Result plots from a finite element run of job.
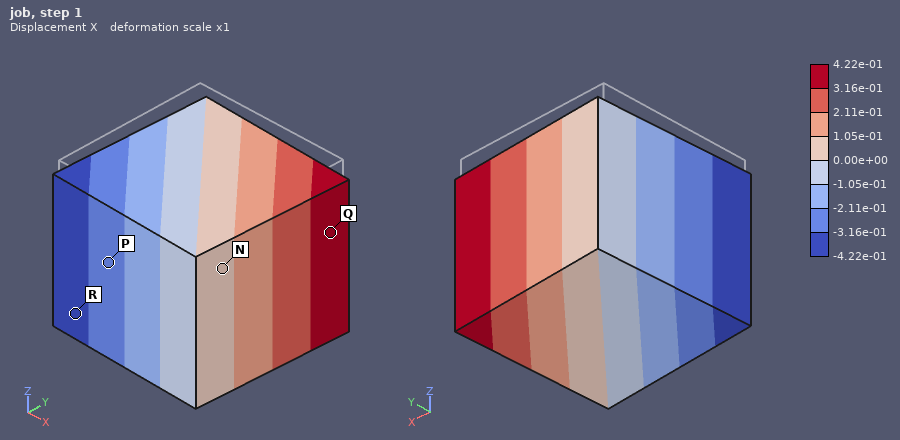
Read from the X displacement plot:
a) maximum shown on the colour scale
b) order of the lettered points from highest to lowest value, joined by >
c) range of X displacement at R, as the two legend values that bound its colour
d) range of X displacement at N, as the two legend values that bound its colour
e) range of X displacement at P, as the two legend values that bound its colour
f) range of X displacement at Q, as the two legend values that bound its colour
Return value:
4.22e-01
Q > N > P > R
-4.22e-01 to -3.16e-01
0.00e+00 to 1.05e-01
-3.16e-01 to -2.11e-01
3.16e-01 to 4.22e-01
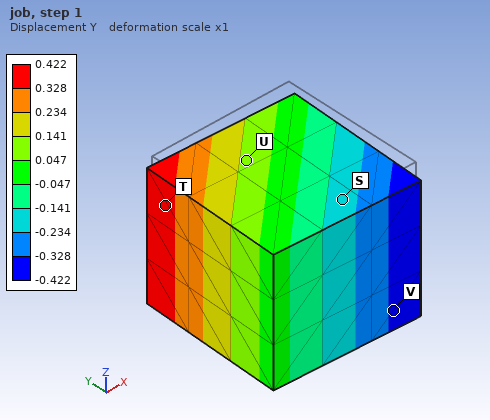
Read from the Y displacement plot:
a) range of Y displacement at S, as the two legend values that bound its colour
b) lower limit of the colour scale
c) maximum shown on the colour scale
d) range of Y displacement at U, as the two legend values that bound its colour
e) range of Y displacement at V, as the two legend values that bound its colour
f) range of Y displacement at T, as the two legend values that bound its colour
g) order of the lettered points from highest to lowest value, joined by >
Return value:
-0.234 to -0.141
-0.422
0.422
0.047 to 0.141
-0.422 to -0.328
0.328 to 0.422
T > U > S > V
